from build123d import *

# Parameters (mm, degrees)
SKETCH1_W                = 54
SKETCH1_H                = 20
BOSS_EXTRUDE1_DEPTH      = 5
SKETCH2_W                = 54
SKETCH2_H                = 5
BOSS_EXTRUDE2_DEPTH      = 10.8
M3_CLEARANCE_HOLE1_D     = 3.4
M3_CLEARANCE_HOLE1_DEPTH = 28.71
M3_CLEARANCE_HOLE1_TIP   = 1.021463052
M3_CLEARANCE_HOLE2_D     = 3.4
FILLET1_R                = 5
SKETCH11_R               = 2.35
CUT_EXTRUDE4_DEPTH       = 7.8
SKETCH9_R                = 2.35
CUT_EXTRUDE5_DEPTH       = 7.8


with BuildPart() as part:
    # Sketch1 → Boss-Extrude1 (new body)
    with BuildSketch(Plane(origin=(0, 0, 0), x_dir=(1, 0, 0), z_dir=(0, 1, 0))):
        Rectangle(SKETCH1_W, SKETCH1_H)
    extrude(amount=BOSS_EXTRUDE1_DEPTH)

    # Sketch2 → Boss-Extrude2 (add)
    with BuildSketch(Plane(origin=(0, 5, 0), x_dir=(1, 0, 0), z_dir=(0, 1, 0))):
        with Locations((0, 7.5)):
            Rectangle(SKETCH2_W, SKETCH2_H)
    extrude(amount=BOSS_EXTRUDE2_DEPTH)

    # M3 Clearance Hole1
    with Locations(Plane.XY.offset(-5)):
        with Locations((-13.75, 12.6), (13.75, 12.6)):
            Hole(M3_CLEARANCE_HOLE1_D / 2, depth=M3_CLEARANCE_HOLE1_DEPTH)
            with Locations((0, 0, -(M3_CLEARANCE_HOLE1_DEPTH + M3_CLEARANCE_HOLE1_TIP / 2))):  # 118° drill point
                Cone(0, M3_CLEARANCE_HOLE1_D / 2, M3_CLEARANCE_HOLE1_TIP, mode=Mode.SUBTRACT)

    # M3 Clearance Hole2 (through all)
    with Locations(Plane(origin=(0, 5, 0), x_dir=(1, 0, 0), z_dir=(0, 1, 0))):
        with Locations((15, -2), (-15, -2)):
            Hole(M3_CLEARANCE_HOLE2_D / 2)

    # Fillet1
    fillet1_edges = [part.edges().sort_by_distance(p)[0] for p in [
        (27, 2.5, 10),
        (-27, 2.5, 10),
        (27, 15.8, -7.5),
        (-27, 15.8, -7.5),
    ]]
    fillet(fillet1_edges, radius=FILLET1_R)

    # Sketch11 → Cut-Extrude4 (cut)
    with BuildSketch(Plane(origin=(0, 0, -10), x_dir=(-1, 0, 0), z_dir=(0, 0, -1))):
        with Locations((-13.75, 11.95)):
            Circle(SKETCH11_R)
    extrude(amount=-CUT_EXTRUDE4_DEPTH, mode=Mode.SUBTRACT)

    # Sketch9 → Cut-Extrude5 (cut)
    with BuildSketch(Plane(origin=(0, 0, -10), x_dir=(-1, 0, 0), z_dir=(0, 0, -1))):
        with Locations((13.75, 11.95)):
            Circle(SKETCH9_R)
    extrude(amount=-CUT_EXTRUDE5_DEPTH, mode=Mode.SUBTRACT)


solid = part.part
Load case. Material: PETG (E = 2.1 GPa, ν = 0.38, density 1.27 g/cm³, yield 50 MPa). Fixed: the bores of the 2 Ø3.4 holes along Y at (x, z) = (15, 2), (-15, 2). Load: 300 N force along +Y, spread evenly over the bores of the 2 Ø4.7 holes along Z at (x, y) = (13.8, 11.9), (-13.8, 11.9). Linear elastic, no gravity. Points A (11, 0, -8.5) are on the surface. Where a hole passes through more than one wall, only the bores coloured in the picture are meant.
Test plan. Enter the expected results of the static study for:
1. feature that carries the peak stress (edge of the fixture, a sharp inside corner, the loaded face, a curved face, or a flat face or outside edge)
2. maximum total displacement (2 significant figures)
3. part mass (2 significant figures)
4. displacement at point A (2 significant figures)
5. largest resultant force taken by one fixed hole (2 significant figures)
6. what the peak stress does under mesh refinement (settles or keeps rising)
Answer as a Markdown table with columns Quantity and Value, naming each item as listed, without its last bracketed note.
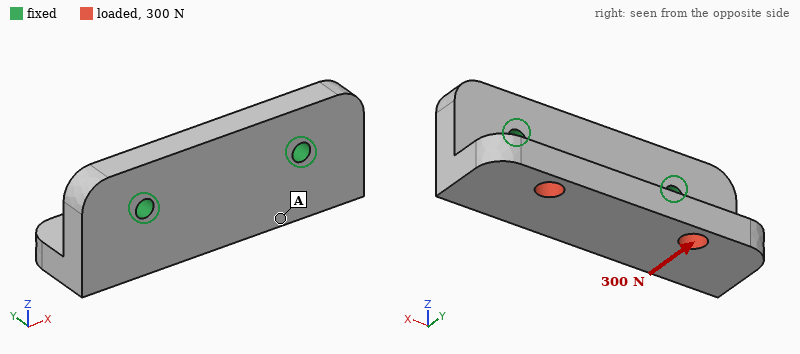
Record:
| Quantity | Value |
|---|---|
| feature that carries the peak stress | edge of the fixture |
| maximum total displacement | 0.31 mm |
| part mass | 10 g |
| displacement at point A | 0.17 mm |
| largest resultant force taken by one fixed hole | 150 N |
| what the peak stress does under mesh refinement | keeps rising |
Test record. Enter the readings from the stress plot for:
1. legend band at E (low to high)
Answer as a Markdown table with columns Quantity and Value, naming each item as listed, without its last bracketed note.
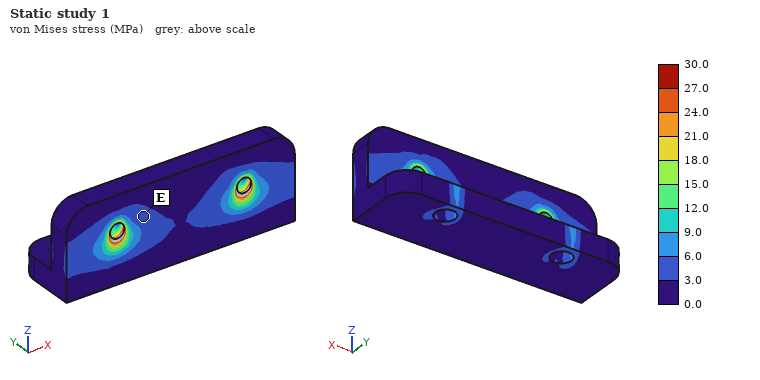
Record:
| Quantity | Value |
|---|---|
| legend band at E | 3.0 to 6.0 MPa |
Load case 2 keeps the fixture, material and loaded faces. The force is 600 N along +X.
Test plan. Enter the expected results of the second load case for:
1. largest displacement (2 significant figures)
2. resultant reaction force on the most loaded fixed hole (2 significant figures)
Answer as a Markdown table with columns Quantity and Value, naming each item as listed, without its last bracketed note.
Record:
| Quantity | Value |
|---|---|
| largest displacement | 0.30 mm |
| resultant reaction force on the most loaded fixed hole | 380 N |
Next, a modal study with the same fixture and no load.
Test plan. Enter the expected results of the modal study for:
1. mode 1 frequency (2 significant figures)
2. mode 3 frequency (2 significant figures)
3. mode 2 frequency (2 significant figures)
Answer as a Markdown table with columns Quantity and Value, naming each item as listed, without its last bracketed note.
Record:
| Quantity | Value |
|---|---|
| mode 1 frequency | 2300 Hz |
| mode 3 frequency | 5200 Hz |
| mode 2 frequency | 3000 Hz |
